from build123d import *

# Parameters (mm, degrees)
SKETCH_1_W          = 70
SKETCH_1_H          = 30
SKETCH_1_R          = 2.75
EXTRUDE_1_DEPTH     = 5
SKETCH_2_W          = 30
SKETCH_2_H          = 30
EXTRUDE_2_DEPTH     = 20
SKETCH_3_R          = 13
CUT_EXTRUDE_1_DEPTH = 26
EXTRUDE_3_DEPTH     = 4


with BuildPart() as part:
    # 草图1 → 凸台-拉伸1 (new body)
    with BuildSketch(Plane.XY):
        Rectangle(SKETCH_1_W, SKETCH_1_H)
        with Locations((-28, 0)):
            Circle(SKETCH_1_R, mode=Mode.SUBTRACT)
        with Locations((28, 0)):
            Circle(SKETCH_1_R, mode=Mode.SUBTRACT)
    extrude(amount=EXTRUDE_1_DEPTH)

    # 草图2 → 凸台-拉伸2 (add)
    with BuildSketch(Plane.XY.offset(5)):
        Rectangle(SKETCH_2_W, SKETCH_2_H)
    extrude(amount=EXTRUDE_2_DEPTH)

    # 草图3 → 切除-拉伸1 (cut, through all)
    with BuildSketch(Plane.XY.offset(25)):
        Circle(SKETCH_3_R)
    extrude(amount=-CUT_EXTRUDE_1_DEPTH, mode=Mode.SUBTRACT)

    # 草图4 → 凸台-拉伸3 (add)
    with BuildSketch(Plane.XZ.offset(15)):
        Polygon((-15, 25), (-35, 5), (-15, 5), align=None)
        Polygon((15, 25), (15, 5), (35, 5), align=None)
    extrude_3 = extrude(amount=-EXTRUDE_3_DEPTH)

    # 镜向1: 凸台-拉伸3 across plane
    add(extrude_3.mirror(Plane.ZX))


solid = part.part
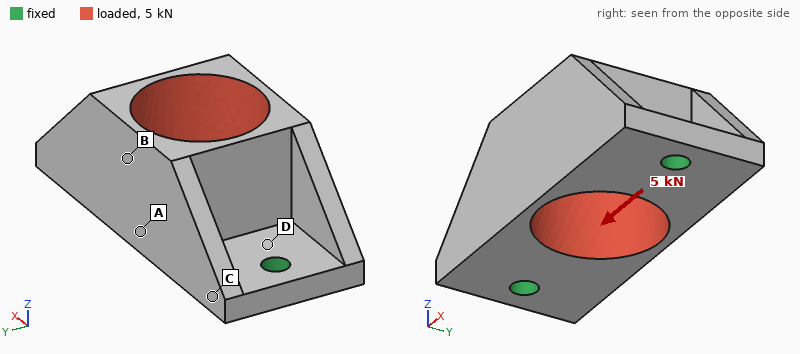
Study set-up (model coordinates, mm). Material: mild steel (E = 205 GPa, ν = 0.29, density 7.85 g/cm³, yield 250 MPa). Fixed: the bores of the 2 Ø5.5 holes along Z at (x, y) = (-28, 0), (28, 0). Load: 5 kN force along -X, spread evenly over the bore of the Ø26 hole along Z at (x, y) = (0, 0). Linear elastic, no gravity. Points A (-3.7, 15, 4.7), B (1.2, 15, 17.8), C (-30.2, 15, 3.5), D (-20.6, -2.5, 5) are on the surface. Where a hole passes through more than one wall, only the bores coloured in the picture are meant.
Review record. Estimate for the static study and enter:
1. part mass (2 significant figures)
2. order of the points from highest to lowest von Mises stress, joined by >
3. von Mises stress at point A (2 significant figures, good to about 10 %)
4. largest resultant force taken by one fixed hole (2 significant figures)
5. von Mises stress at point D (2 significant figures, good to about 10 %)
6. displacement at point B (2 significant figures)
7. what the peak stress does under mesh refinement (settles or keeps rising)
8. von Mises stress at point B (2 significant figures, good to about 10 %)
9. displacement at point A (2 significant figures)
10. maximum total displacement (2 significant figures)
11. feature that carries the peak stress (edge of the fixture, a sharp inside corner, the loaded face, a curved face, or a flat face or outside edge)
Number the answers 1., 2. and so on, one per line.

1. 140 g
2. D > B > A > C
3. 15 MPa
4. 2.7 kN
5. 37 MPa
6. 5.5 µm
7. keeps rising
8. 25 MPa
9. 3.0 µm
10. 10 µm
11. edge of the fixture
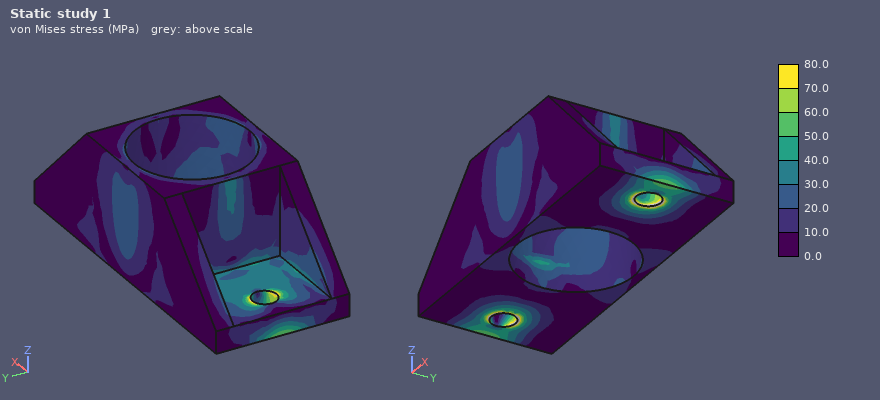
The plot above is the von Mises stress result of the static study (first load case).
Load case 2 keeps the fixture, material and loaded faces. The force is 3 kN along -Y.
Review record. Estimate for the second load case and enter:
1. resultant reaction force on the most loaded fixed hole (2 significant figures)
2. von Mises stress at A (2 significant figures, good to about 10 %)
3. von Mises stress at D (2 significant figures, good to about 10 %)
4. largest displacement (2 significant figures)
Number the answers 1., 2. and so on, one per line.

1. 1.5 kN
2. 41 MPa
3. 67 MPa
4. 43 µm
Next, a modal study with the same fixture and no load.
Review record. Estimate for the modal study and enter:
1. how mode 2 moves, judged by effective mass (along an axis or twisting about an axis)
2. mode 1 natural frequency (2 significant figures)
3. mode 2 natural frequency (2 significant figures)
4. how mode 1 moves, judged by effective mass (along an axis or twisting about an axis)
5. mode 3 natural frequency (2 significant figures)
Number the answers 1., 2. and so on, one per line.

1. along Z
2. 4700 Hz
3. 9400 Hz
4. along Y
5. 10 kHz
